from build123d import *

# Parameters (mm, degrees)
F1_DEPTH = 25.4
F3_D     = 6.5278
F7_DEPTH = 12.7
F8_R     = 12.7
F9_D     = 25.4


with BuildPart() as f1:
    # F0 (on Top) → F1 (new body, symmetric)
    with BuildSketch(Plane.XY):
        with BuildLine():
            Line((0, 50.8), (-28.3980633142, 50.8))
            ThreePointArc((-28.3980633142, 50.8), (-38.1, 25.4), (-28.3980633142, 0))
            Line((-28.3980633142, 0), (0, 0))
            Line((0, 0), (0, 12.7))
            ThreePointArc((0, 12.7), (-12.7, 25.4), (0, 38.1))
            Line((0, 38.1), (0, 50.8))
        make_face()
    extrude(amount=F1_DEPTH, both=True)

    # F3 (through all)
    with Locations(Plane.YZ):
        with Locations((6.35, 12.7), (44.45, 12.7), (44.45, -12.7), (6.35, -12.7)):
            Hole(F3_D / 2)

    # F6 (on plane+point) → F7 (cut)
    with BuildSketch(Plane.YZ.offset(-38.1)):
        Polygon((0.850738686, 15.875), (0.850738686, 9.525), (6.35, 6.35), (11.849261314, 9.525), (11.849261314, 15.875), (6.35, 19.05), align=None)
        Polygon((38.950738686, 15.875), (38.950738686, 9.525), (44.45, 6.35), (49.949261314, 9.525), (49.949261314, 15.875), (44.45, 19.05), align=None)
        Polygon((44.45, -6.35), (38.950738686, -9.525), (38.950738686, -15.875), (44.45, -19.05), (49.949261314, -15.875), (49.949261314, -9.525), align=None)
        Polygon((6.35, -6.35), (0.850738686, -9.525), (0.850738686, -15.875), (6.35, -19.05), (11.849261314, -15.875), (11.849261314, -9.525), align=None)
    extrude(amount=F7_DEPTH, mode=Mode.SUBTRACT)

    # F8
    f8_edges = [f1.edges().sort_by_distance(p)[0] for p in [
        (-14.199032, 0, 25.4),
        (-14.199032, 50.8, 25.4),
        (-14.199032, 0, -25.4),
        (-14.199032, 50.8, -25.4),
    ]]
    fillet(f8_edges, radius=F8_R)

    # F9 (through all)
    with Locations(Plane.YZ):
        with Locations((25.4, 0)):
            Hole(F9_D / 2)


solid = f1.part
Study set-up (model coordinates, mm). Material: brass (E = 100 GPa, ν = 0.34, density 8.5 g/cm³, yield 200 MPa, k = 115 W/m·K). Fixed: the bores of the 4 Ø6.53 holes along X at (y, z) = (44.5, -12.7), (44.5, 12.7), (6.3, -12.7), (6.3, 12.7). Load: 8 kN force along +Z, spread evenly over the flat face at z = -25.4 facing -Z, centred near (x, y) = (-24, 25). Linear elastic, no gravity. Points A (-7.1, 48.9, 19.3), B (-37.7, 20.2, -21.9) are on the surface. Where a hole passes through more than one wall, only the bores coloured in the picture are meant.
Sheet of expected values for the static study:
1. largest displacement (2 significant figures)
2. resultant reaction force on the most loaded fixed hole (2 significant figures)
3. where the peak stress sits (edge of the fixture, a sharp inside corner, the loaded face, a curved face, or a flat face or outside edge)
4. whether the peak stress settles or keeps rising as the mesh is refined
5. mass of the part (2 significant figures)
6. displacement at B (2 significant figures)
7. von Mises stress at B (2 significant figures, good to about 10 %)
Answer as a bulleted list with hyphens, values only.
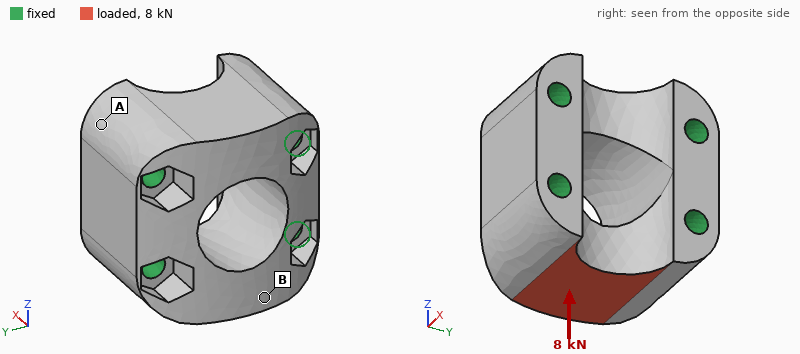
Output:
- 11 µm
- 3.4 kN
- edge of the fixture
- keeps rising
- 450 g
- 9.3 µm
- 13 MPa
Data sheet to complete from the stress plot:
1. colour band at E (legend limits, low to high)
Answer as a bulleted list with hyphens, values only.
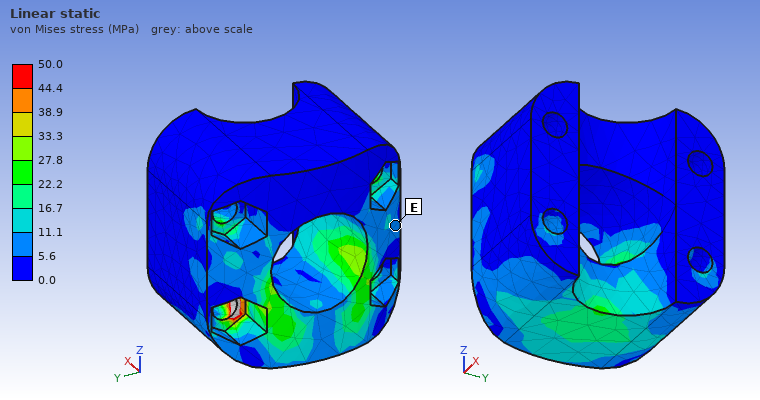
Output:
- 5.6 to 11.1 MPa
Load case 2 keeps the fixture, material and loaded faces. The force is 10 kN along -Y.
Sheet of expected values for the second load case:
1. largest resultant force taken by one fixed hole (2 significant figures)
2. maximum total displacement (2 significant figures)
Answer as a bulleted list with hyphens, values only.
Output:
- 5.6 kN
- 7.4 µm
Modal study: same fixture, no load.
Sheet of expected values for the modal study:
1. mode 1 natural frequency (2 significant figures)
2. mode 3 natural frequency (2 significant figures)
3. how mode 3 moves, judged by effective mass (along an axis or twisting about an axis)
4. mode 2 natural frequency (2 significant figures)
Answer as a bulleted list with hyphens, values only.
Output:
- 17 kHz
- 24 kHz
- along Y
- 17 kHz
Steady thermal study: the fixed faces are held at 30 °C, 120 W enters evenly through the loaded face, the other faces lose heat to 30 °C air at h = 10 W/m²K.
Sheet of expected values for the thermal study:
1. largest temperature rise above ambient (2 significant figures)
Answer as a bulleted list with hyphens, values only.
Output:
- 30 K
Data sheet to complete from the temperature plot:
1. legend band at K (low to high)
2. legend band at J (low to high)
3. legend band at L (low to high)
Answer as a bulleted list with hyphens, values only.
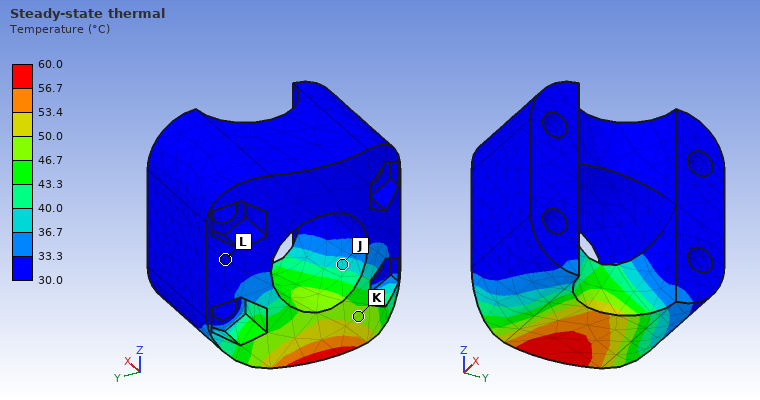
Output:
- 46.7 to 50.0 °C
- 36.7 to 40.0 °C
- 30.0 to 33.3 °C
